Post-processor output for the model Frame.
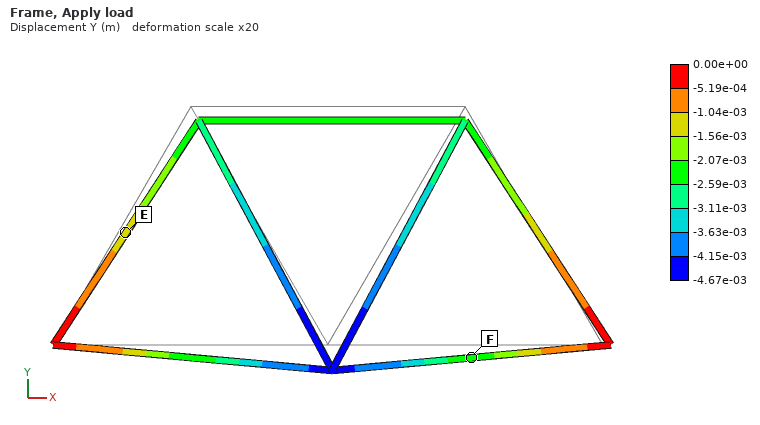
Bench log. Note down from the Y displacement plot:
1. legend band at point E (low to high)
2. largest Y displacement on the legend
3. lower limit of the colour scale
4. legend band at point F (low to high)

-1.56e-03 to -1.04e-03 m
0.00e+00 m
-4.67e-03 m
-2.59e-03 to -2.07e-03 m
